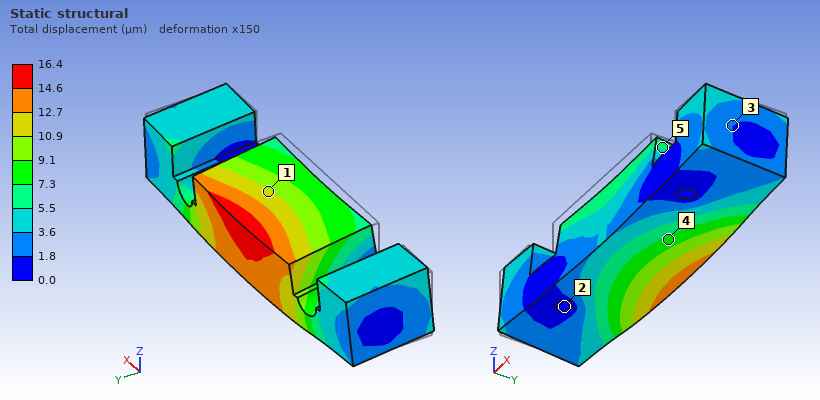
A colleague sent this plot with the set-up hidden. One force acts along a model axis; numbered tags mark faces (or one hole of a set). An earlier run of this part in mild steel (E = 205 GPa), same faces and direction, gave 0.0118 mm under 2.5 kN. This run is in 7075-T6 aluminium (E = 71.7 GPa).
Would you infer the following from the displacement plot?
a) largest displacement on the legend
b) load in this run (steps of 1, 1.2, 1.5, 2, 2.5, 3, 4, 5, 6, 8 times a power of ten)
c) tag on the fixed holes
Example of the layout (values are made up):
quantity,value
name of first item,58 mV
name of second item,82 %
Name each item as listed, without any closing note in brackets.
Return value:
quantity,value
largest displacement on the legend,16.4 µm
load in this run,1.2 kN
tag on the fixed holes,2
